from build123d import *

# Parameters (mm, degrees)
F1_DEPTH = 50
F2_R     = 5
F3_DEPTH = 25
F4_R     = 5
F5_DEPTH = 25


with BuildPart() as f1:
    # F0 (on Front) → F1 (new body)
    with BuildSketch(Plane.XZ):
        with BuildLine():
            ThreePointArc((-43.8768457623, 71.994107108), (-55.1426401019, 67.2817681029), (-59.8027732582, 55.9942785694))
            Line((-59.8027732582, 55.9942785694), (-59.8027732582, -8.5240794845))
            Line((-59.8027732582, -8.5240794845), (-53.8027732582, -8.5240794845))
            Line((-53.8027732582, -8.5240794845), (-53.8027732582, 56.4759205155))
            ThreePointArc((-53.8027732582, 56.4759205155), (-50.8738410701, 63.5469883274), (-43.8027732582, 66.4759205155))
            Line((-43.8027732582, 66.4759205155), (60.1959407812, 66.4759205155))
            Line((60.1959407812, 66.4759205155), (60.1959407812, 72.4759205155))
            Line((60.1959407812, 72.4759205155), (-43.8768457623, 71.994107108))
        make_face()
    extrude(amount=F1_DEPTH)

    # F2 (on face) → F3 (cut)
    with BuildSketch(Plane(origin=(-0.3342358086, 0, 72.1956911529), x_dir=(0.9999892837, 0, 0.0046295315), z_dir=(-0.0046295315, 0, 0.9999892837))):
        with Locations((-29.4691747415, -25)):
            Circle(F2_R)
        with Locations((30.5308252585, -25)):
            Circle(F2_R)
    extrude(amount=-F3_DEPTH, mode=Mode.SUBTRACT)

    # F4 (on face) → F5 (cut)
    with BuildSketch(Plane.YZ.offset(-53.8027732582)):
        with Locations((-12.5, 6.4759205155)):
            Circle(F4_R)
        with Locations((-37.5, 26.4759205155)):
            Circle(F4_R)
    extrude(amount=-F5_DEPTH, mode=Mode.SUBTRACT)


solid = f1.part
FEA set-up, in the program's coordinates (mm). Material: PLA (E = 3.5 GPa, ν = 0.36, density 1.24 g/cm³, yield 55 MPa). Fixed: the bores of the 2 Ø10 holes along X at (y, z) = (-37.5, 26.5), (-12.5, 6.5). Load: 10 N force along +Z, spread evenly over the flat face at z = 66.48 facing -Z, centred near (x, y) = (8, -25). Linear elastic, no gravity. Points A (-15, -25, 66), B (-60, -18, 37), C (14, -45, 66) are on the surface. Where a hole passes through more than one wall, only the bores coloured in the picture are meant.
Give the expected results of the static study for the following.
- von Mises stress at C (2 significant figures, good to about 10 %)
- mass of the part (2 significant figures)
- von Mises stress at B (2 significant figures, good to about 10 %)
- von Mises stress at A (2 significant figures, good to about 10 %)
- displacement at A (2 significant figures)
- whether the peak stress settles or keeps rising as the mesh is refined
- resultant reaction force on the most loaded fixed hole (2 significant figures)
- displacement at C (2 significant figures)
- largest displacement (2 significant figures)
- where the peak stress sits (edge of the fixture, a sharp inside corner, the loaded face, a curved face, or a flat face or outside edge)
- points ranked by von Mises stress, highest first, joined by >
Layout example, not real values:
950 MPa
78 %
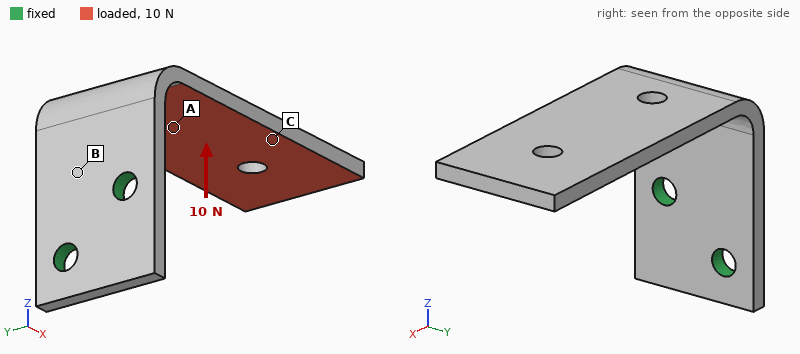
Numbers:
0.39 MPa
66 g
1.7 MPa
0.85 MPa
0.50 mm
keeps rising
11 N
0.94 mm
1.7 mm
edge of the fixture
B > A > C
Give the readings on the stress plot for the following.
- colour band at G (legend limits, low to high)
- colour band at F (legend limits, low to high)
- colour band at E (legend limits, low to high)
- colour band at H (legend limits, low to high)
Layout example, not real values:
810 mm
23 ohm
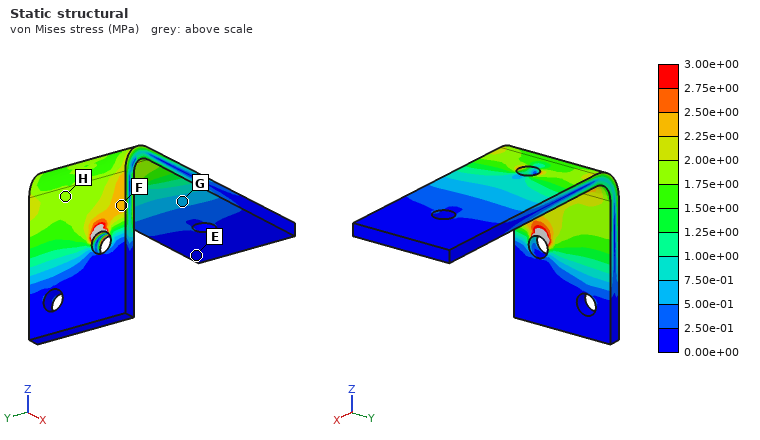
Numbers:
5.00e-01 to 7.50e-01 MPa
2.25e+00 to 2.50e+00 MPa
0.00e+00 to 2.50e-01 MPa
1.75e+00 to 2.00e+00 MPa
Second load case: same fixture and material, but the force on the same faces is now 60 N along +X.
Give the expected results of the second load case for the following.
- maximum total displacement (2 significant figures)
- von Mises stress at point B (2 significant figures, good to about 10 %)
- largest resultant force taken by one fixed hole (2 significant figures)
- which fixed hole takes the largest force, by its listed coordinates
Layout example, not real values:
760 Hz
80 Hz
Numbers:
1.6 mm
4.4 MPa
74 N
(-37.5, 26.5)
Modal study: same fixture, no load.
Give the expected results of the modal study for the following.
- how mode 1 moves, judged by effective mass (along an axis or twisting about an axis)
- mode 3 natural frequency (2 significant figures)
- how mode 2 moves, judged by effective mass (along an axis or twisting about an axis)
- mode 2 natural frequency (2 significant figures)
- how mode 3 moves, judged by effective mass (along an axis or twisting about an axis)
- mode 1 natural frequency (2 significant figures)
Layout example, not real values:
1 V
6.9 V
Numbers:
along Z
340 Hz
along Y
130 Hz
along X
76 Hz
